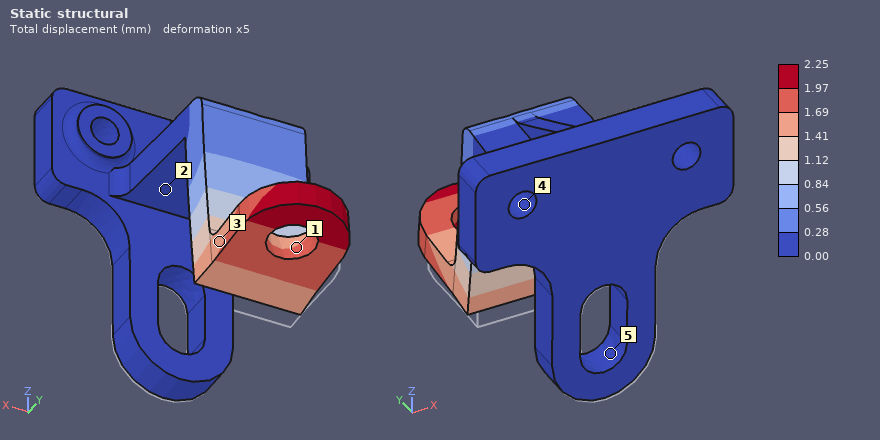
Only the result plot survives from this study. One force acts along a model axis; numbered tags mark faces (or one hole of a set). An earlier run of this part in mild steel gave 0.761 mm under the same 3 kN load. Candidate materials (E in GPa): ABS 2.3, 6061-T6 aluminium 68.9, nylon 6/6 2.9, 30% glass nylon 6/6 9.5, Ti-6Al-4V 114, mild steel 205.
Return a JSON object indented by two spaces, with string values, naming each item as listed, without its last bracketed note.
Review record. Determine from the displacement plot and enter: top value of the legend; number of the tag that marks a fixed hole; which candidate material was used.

{
  "top value of the legend": "2.25 mm",
  "number of the tag that marks a fixed hole": "4",
  "which candidate material was used": "6061-T6 aluminium"
}
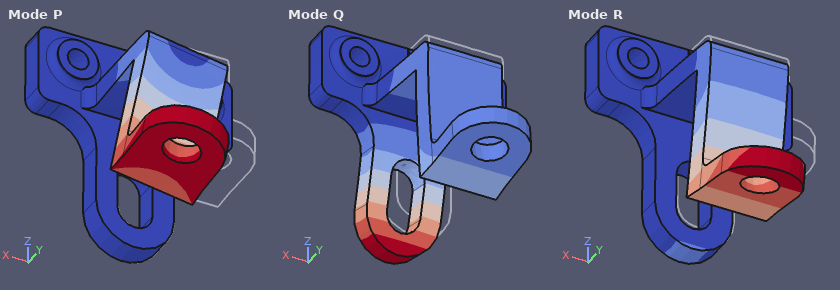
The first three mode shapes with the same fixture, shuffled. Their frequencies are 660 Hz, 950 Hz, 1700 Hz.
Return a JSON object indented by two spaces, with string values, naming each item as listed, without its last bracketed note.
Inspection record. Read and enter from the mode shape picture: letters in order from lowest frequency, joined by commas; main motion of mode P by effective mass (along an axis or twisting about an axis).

{
  "letters in order from lowest frequency, joined by commas": "R, P, Q",
  "main motion of mode P by effective mass": "along X"
}
